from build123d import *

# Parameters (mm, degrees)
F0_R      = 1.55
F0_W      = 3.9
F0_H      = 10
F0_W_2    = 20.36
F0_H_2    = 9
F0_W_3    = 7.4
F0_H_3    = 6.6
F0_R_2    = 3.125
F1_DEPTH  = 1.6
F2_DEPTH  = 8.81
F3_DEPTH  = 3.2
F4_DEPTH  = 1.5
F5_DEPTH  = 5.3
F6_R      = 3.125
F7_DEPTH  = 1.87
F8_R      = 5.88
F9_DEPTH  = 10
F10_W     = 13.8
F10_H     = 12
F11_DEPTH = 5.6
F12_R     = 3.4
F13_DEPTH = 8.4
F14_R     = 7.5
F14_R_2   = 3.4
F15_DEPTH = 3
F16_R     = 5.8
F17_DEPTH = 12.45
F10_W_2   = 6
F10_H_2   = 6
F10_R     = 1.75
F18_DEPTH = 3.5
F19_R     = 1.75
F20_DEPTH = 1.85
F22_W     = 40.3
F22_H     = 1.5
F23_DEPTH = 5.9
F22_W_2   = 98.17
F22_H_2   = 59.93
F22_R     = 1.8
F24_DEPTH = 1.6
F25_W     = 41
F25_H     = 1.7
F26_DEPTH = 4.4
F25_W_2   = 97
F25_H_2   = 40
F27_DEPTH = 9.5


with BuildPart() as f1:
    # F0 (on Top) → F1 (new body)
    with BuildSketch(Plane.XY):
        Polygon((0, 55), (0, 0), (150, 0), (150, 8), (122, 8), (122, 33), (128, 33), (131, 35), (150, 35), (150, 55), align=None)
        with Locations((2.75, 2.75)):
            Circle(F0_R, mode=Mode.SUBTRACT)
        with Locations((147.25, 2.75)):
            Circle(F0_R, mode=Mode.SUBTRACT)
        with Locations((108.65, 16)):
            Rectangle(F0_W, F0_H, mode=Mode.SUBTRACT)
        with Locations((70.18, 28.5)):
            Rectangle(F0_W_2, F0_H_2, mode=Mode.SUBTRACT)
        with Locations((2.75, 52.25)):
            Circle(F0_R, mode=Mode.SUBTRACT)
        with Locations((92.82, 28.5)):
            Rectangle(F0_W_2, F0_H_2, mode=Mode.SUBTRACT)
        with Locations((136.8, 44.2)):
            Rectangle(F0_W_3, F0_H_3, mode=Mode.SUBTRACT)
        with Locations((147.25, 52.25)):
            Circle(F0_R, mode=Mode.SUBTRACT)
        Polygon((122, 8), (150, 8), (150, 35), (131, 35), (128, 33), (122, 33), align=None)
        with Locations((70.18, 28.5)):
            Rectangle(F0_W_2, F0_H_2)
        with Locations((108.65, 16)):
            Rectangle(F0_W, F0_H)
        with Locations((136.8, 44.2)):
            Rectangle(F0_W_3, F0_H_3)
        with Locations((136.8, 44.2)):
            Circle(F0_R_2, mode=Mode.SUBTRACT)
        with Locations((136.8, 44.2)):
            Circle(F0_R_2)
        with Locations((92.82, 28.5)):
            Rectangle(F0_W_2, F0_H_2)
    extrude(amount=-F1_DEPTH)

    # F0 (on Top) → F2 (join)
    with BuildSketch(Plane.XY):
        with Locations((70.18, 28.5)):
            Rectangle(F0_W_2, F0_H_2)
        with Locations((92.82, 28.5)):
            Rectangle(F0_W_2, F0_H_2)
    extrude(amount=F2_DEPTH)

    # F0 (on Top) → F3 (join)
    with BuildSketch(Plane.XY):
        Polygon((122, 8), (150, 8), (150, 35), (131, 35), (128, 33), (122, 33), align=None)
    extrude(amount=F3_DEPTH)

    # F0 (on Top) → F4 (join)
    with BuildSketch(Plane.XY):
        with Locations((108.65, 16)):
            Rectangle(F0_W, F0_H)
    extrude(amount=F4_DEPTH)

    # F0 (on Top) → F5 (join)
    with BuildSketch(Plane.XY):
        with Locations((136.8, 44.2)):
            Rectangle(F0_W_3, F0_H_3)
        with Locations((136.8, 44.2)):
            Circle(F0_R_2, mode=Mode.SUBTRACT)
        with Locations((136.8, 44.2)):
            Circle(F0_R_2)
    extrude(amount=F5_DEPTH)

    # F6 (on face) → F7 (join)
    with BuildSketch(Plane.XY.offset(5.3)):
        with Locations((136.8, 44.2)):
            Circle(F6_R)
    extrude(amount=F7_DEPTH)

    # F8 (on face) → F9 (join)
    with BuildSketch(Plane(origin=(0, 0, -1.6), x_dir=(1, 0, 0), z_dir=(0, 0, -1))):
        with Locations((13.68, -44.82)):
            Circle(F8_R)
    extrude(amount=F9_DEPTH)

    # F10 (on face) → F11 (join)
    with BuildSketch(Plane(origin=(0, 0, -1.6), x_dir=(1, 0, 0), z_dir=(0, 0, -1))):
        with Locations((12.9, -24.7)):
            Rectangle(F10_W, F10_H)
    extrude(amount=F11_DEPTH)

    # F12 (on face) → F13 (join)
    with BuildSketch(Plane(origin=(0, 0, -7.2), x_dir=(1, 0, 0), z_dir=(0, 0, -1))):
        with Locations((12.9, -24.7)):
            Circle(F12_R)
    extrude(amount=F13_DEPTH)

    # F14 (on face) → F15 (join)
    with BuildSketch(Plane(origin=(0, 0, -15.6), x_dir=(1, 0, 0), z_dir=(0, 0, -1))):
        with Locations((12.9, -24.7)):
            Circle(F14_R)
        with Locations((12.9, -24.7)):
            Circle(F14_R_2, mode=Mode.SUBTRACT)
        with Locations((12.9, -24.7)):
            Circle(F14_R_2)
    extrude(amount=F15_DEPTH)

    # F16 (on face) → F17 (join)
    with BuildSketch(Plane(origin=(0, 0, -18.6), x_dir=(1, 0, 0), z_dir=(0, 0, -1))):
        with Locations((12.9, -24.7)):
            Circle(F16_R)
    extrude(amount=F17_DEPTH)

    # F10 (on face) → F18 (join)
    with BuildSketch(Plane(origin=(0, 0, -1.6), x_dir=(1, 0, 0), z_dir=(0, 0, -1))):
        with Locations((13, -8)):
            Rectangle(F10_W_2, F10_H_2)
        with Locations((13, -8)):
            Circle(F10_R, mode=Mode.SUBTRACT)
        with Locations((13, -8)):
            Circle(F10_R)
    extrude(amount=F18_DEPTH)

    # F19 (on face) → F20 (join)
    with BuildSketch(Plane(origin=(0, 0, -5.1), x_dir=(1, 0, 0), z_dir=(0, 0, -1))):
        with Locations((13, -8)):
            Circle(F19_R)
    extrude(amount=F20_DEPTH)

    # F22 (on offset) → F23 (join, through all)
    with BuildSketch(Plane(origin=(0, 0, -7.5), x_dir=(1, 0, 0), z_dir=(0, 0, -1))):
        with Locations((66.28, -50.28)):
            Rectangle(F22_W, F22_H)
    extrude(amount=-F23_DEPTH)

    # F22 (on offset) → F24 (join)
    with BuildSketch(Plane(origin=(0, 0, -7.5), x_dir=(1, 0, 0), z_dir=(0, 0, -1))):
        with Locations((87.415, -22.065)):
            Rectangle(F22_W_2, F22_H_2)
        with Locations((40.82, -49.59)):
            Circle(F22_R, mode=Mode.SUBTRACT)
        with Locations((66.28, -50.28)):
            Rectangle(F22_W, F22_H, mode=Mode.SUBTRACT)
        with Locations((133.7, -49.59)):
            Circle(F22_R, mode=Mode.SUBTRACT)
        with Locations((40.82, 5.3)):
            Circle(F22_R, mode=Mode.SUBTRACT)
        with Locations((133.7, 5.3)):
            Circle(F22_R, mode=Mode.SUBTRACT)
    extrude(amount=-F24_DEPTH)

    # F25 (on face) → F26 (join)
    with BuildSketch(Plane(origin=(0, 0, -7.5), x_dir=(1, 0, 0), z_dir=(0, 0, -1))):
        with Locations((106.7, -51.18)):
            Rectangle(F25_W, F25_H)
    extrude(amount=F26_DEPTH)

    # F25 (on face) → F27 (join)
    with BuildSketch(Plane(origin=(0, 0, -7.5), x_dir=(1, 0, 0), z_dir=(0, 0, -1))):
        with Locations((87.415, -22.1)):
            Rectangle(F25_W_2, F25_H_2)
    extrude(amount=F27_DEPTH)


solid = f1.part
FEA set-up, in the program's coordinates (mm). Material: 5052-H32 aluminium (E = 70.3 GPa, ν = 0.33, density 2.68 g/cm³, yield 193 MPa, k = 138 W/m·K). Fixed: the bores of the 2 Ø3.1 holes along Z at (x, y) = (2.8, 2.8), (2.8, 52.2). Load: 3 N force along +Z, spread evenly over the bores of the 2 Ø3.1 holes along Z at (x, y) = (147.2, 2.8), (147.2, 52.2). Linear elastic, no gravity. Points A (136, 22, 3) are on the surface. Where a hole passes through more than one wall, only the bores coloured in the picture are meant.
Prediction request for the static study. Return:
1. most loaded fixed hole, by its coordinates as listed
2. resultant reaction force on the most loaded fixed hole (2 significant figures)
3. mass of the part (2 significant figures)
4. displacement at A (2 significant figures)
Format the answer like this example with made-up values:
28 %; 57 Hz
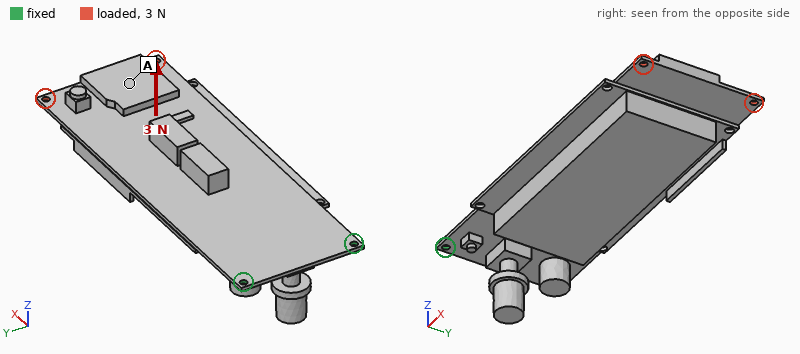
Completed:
(2.8, 2.8); 2.3 N; 190 g; 1.6 mm
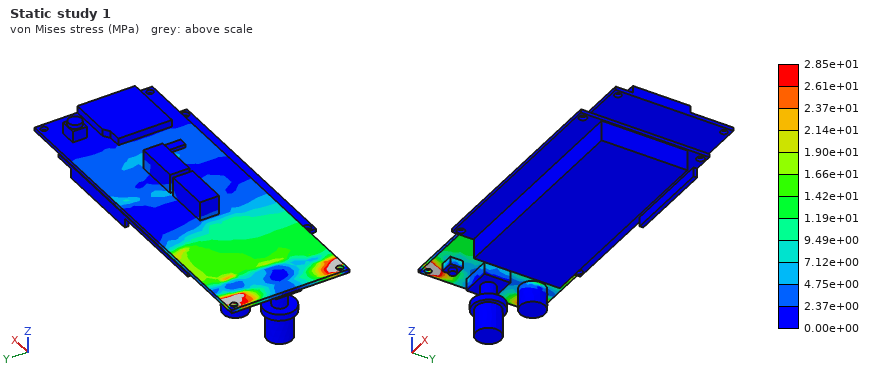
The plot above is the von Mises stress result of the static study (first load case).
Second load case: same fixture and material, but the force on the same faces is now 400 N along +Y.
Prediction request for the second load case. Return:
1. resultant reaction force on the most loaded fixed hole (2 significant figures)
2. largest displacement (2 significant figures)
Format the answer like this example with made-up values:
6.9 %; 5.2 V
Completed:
1.2 kN; 0.36 mm
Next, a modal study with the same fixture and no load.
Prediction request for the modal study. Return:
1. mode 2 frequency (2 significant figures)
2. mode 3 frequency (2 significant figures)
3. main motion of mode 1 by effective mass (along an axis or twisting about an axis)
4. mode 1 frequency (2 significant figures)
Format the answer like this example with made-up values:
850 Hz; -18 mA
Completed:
120 Hz; 230 Hz; along Z; 27 Hz
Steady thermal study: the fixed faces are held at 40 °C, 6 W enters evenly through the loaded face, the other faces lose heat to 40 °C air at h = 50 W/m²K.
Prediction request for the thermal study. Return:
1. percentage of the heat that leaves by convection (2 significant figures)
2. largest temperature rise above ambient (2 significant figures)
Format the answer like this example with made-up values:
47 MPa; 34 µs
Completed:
96 %; 30 K
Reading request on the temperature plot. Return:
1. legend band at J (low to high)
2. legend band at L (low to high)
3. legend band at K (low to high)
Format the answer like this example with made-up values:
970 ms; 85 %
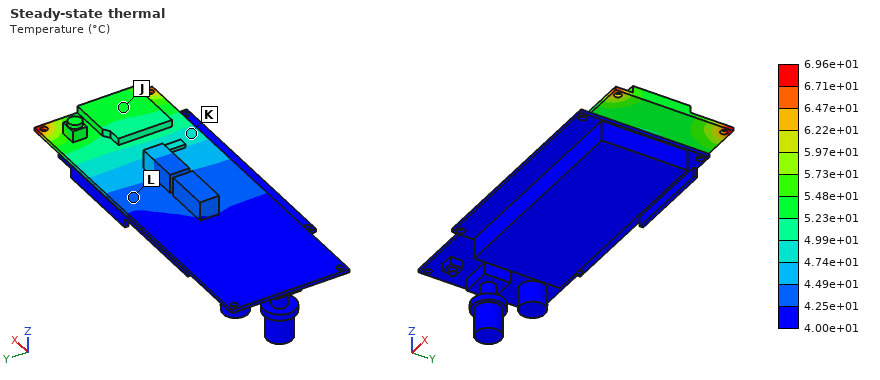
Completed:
5.23e+01 to 5.48e+01 °C; 4.25e+01 to 4.49e+01 °C; 4.74e+01 to 4.99e+01 °C
